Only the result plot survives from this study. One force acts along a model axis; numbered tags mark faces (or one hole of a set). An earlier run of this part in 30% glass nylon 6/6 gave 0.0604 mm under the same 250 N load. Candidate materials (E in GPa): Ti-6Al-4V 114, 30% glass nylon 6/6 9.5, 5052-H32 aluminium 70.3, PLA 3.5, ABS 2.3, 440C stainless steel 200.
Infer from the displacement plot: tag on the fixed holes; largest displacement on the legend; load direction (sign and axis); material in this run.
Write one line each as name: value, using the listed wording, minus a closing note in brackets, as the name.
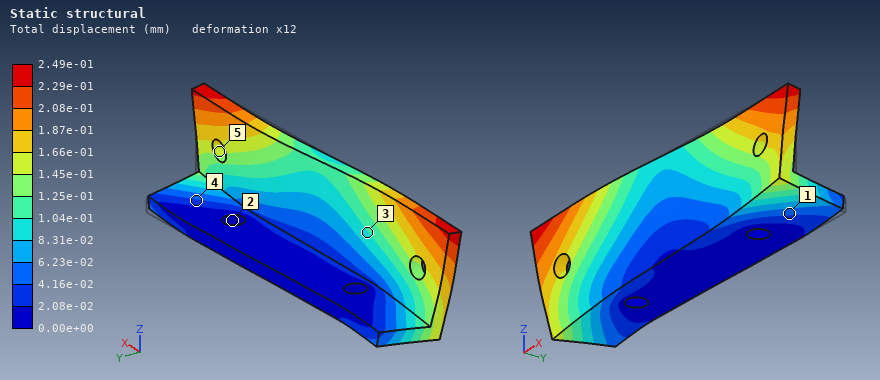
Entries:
tag on the fixed holes: 2
largest displacement on the legend: 2.49e-01 mm
load direction: -X
material in this run: ABS
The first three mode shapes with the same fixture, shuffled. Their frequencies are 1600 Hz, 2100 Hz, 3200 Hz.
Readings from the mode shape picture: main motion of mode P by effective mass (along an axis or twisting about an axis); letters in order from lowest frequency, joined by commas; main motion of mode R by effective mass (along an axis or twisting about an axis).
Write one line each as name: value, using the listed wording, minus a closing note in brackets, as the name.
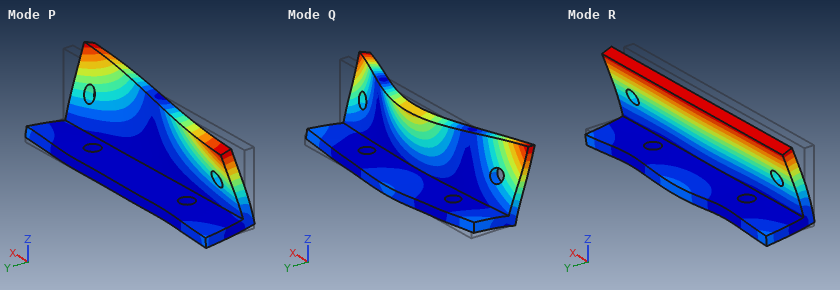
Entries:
main motion of mode P by effective mass: twisting about Z
letters in order from lowest frequency, joined by commas: R, P, Q
main motion of mode R by effective mass: along Y
